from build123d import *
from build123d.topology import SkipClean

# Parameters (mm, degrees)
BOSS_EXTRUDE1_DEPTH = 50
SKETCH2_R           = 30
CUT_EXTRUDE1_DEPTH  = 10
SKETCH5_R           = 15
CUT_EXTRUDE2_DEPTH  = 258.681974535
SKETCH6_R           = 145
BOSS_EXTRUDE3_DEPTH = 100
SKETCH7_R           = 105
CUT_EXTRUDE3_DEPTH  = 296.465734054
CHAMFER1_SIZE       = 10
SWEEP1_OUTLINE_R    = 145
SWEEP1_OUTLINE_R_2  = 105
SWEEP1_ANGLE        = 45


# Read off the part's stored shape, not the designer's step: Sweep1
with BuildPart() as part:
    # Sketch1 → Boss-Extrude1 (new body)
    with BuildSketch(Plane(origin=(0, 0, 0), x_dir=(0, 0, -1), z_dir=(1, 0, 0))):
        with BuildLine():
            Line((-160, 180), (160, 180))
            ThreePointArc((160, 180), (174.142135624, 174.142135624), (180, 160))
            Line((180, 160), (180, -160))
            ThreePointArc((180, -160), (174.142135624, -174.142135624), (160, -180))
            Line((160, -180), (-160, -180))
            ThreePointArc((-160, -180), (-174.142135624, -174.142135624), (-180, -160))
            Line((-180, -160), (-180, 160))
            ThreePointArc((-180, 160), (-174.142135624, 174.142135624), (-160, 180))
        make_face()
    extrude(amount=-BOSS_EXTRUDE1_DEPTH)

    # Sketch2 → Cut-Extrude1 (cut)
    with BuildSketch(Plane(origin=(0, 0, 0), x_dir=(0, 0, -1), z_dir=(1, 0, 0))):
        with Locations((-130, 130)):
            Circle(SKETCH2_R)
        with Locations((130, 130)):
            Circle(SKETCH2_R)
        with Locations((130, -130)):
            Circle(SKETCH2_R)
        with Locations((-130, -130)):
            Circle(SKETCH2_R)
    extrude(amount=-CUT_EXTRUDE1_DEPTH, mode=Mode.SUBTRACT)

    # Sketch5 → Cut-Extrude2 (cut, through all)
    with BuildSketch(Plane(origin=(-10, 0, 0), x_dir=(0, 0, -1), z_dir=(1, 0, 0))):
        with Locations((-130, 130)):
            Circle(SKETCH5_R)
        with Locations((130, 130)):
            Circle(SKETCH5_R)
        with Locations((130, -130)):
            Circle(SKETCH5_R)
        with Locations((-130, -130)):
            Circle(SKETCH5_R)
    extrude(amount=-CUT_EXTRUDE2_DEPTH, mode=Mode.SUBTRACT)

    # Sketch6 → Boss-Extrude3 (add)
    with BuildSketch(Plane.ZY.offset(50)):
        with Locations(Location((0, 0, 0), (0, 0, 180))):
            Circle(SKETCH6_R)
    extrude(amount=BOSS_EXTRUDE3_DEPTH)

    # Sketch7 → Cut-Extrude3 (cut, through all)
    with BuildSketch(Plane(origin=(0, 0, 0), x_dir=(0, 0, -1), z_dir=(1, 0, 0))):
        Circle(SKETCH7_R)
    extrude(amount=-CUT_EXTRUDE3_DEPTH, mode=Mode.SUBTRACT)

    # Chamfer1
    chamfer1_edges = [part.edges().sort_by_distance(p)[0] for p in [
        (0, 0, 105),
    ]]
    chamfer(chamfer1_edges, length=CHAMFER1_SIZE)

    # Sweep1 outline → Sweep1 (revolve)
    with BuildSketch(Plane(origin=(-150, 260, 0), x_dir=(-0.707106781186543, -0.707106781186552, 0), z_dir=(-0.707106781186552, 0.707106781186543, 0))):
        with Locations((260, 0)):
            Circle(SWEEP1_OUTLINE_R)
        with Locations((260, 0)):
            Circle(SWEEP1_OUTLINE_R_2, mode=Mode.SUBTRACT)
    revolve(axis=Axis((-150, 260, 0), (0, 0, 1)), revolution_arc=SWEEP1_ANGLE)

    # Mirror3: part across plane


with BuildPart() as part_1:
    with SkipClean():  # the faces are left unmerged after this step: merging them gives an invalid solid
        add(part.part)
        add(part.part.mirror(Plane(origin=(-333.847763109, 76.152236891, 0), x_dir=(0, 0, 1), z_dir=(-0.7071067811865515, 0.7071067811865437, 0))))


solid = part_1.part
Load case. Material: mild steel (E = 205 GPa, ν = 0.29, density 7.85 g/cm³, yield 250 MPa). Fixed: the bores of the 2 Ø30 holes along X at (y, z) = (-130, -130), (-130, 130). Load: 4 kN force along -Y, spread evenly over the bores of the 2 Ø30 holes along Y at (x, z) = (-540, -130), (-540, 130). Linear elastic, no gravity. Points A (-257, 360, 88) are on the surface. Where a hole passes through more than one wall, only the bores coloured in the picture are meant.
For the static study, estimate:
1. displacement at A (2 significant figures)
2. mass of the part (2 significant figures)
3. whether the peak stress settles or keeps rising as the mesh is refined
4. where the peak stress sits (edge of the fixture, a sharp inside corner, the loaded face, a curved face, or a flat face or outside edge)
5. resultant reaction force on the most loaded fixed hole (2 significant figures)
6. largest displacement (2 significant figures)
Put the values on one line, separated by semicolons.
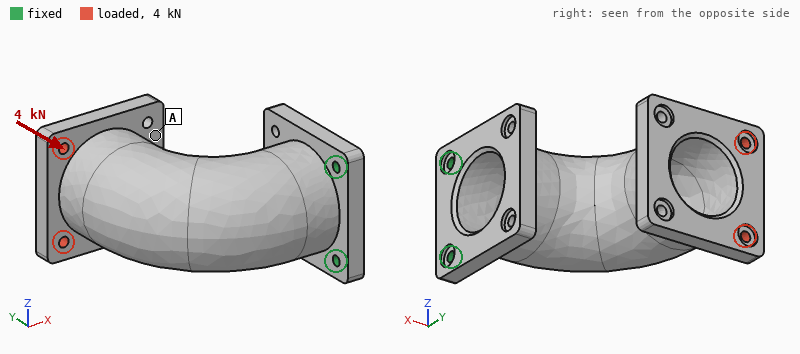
0.15 mm; 220 kg; keeps rising; edge of the fixture; 2.0 kN; 0.22 mm
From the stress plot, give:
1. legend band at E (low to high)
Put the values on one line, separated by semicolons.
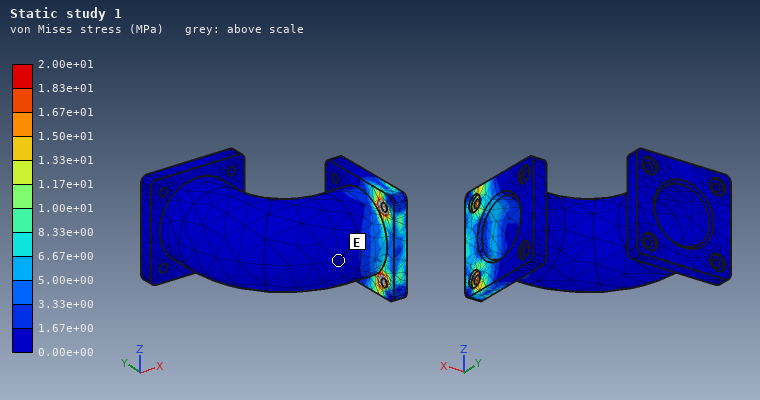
0.00e+00 to 1.67e+00 MPa
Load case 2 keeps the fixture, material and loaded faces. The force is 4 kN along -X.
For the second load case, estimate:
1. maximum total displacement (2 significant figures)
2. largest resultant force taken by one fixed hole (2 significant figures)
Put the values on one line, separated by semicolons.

0.21 mm; 2.0 kN
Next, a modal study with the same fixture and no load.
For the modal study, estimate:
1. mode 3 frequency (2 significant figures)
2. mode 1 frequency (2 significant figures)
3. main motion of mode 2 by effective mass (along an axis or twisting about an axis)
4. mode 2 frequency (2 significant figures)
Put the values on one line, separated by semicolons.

550 Hz; 69 Hz; along Z; 220 Hz
